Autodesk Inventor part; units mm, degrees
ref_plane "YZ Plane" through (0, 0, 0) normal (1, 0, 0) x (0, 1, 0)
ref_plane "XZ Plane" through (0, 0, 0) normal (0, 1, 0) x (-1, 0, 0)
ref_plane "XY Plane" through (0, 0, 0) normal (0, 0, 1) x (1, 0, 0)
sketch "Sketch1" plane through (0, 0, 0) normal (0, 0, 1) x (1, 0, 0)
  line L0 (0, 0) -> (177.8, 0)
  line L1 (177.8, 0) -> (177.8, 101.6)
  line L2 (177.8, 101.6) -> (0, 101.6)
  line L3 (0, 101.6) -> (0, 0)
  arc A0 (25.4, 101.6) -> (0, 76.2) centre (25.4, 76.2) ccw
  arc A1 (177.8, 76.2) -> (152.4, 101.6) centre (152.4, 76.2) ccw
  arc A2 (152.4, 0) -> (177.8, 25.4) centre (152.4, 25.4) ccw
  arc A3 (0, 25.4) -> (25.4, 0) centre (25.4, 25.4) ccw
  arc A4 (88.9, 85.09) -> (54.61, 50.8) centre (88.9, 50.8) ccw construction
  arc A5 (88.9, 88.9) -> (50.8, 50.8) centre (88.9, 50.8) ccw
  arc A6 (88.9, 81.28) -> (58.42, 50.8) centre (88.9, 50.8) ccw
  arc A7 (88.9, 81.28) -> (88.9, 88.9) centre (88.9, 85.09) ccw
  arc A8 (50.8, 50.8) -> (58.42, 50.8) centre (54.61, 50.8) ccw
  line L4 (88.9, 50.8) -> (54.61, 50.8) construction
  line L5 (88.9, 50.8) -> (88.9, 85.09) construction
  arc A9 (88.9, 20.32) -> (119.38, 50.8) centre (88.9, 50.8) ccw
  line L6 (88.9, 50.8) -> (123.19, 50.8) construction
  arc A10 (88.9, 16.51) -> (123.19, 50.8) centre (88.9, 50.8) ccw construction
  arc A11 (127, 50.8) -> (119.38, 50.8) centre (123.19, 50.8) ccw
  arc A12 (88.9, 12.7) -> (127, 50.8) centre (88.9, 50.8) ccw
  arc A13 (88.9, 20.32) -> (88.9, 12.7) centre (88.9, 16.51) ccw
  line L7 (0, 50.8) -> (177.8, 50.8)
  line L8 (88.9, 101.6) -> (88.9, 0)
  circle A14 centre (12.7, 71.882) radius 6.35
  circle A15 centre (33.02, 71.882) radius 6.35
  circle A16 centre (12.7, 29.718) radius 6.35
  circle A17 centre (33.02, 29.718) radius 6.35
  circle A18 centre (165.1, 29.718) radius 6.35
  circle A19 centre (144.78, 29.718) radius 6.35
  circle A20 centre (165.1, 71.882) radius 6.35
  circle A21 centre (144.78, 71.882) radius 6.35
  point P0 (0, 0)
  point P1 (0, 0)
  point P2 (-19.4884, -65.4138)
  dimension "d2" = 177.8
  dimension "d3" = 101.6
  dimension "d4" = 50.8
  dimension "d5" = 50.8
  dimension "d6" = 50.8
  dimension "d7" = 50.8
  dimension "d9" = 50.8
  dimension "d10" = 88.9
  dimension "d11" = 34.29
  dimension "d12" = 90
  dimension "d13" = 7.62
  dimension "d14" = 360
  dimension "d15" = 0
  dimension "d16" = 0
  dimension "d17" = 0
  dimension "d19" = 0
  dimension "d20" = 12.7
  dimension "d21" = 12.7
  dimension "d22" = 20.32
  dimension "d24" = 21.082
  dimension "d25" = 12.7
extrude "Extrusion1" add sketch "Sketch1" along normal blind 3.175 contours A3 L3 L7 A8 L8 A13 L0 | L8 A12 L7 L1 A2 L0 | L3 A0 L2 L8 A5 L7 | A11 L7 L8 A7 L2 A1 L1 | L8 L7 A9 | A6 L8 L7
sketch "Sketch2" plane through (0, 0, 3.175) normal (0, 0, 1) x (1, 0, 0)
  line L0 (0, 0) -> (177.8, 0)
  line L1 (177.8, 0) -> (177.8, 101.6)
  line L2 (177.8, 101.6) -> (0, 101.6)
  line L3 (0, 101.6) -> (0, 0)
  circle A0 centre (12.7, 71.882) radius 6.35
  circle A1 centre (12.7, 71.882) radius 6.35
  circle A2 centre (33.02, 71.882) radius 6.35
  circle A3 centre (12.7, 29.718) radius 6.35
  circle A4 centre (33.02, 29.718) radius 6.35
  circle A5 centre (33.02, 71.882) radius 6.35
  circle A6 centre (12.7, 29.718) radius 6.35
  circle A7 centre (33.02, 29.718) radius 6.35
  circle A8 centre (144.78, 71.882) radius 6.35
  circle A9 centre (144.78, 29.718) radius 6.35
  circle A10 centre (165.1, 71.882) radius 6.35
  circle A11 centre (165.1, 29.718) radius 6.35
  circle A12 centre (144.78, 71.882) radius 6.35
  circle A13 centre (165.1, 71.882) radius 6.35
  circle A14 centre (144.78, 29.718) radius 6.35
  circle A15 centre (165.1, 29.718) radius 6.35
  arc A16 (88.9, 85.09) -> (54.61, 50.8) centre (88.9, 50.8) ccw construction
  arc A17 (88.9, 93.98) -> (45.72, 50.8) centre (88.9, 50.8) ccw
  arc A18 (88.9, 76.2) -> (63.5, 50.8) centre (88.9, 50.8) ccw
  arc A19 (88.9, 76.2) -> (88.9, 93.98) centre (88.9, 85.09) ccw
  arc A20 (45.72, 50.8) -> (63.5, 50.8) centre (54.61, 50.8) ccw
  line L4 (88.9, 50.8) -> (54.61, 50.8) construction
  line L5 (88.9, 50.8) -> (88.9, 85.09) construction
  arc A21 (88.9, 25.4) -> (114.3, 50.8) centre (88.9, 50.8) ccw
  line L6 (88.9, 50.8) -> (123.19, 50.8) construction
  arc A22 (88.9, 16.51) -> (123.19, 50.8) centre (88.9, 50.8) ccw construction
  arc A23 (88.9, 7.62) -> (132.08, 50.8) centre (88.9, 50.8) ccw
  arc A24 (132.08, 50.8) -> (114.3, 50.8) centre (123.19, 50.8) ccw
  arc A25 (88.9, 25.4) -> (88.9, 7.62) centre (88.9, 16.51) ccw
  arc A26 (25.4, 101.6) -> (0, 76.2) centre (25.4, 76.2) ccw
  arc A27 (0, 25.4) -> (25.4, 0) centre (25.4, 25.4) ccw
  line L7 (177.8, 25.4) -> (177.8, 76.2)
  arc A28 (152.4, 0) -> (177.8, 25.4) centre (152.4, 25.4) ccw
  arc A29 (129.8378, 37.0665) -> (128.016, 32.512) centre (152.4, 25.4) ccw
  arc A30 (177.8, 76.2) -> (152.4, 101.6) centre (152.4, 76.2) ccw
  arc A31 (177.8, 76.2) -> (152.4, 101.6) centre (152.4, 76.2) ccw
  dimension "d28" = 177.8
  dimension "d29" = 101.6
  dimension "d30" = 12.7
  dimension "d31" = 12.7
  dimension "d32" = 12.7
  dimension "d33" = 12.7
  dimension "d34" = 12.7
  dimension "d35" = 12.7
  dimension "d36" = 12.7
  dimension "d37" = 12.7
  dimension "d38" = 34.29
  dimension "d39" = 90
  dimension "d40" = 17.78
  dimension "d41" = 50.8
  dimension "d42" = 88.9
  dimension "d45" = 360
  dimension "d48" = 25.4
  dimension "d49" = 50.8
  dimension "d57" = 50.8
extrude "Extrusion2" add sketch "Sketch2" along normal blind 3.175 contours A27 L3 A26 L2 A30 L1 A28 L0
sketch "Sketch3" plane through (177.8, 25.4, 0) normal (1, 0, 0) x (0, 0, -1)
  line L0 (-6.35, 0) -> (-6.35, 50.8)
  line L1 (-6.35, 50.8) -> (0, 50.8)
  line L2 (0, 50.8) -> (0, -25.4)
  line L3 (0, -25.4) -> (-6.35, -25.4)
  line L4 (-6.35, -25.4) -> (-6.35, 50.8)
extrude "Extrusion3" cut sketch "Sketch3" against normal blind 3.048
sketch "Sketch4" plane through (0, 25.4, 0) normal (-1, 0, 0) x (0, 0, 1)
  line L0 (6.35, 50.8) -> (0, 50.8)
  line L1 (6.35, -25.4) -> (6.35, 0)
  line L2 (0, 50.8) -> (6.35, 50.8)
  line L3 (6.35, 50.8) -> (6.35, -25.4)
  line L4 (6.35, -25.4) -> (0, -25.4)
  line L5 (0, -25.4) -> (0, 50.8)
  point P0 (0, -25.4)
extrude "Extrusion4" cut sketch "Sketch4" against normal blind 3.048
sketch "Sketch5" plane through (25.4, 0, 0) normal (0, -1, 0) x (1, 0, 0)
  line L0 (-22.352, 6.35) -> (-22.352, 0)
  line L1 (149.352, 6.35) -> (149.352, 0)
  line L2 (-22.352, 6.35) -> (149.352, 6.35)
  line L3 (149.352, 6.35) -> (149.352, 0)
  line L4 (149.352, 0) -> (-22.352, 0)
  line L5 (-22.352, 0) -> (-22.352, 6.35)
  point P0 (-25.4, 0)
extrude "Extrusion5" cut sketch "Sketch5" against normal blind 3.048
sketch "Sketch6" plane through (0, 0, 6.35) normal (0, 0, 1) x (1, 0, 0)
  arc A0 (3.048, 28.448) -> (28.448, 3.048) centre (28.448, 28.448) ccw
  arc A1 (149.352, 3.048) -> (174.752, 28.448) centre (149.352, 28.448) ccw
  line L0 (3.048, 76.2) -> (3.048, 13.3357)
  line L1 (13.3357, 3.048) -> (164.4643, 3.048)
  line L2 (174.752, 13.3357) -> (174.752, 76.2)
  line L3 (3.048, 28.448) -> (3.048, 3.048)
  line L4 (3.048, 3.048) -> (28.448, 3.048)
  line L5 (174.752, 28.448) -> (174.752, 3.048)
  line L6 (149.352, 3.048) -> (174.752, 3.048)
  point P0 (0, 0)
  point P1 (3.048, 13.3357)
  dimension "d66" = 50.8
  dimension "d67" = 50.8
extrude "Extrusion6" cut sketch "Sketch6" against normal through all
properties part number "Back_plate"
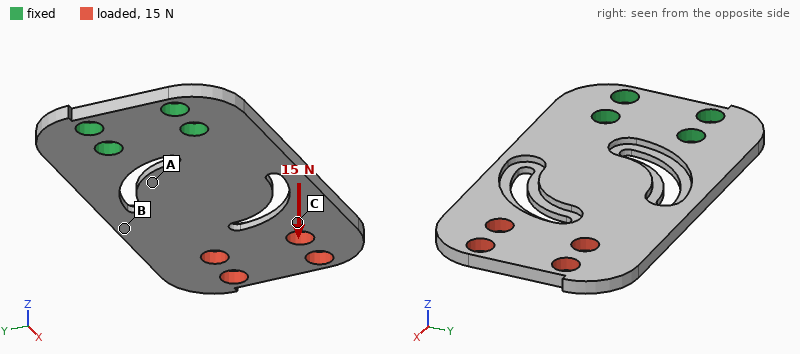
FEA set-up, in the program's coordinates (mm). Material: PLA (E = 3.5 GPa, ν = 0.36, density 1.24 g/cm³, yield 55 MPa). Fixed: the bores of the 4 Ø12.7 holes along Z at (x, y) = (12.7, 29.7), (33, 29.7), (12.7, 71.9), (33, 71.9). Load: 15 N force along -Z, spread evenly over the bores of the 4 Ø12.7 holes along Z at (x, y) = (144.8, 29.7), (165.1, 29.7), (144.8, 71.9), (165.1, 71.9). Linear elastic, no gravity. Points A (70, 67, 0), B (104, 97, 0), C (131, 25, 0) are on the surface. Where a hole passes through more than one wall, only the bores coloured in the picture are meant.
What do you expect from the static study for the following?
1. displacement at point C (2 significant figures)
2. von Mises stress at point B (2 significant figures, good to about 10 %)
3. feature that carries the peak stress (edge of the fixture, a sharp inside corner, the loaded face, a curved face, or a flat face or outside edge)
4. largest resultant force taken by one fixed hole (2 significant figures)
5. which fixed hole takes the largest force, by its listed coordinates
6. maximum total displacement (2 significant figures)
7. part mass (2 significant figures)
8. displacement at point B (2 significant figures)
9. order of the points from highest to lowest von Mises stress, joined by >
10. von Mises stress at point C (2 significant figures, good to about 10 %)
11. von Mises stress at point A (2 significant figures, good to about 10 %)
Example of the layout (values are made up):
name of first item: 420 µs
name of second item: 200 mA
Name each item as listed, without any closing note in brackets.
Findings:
displacement at point C: 1.3 mm
von Mises stress at point B: 1.4 MPa
feature that carries the peak stress: a curved face
largest resultant force taken by one fixed hole: 25 N
which fixed hole takes the largest force, by its listed coordinates: (33, 29.7)
maximum total displacement: 2.3 mm
part mass: 110 g
displacement at point B: 0.63 mm
order of the points from highest to lowest von Mises stress, joined by >: B > A > C
von Mises stress at point C: 0.48 MPa
von Mises stress at point A: 0.96 MPa
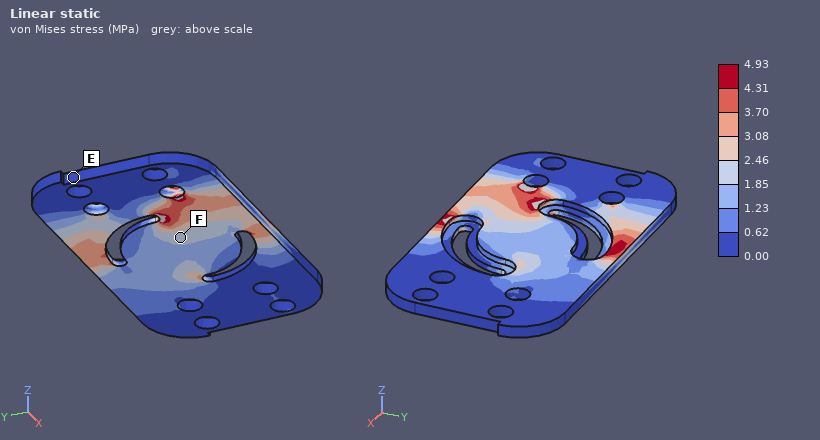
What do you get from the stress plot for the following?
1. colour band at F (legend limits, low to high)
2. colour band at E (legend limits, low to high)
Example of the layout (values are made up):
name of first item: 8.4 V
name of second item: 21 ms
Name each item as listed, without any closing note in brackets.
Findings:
colour band at F: 1.85 to 2.46 MPa
colour band at E: 0.00 to 0.62 MPa
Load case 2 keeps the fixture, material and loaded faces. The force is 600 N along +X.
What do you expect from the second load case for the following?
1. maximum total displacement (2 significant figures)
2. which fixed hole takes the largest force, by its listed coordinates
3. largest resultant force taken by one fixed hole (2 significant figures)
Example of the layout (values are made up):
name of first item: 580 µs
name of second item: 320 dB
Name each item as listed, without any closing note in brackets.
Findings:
maximum total displacement: 0.34 mm
which fixed hole takes the largest force, by its listed coordinates: (33, 29.7)
largest resultant force taken by one fixed hole: 310 N
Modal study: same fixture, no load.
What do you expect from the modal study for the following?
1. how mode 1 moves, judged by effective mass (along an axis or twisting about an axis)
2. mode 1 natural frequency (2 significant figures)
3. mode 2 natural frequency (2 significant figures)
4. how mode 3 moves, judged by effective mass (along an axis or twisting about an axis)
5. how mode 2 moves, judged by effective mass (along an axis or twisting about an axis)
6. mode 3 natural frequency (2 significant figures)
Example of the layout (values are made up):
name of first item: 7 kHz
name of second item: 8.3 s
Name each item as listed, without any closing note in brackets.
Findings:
how mode 1 moves, judged by effective mass: along Z
mode 1 natural frequency: 80 Hz
mode 2 natural frequency: 250 Hz
how mode 3 moves, judged by effective mass: along Z
how mode 2 moves, judged by effective mass: twisting about X
mode 3 natural frequency: 490 Hz
